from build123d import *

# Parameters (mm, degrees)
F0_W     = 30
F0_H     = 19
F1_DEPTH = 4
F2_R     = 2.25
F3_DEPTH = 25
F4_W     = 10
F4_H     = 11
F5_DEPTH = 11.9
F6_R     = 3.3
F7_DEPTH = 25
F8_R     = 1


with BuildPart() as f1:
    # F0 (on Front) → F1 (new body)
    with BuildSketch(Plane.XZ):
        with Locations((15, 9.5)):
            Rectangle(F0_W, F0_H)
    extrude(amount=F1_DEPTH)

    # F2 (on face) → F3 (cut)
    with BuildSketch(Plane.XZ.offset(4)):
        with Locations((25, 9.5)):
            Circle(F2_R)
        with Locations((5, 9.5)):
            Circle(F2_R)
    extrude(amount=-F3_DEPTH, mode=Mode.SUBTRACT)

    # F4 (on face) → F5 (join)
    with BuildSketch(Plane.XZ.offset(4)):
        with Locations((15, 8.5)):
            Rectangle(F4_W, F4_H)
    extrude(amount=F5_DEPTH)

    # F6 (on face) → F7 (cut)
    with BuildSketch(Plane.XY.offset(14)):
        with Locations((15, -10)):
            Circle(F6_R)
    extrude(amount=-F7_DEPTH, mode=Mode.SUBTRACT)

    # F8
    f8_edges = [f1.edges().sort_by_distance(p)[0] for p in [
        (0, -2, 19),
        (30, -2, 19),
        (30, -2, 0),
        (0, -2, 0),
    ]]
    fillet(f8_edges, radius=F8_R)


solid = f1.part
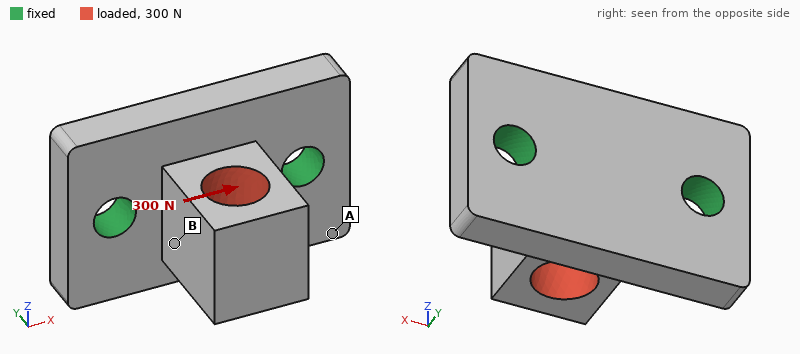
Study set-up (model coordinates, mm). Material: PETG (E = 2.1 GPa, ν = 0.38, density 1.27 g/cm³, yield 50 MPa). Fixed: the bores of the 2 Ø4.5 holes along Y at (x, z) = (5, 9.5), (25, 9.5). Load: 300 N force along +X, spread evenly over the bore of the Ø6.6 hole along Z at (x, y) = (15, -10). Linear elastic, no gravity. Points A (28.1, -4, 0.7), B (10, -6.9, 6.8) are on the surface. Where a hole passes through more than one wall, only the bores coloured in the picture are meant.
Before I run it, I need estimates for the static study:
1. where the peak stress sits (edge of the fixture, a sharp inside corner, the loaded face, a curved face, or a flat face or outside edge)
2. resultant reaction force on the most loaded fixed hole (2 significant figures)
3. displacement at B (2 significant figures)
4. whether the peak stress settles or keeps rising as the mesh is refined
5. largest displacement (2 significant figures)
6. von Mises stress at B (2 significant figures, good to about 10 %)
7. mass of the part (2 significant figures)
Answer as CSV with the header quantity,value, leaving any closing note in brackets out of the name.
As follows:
quantity,value
where the peak stress sits,edge of the fixture
resultant reaction force on the most loaded fixed hole,220 N
displacement at B,0.077 mm
whether the peak stress settles or keeps rising as the mesh is refined,keeps rising
largest displacement,0.26 mm
von Mises stress at B,15 MPa
mass of the part,3.9 g
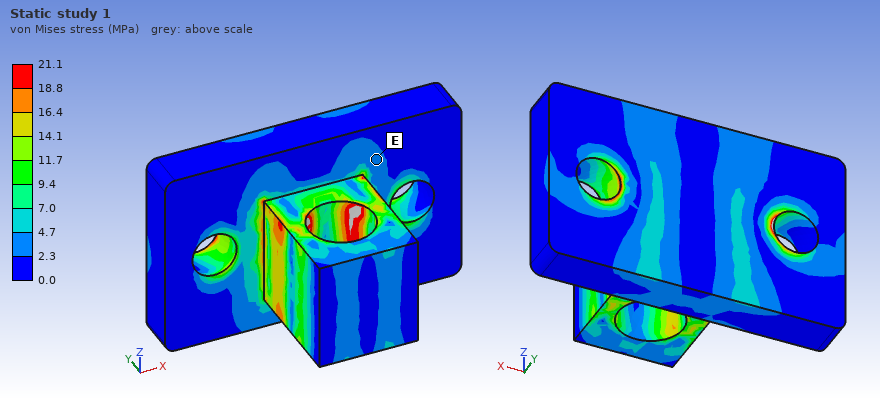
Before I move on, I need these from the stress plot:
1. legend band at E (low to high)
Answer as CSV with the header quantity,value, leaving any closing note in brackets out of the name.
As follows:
quantity,value
legend band at E,2.3 to 4.7 MPa
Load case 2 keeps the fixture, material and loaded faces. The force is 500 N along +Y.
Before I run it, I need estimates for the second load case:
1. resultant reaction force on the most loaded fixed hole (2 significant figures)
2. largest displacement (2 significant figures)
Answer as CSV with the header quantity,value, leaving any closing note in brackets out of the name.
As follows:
quantity,value
resultant reaction force on the most loaded fixed hole,260 N
largest displacement,0.14 mm
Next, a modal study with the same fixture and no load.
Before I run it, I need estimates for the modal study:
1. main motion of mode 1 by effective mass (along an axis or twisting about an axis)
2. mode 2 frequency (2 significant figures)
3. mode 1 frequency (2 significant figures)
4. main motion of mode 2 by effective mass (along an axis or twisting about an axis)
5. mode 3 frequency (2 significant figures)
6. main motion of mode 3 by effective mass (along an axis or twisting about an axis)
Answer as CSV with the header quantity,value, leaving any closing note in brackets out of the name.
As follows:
quantity,value
main motion of mode 1 by effective mass,along Z
mode 2 frequency,5500 Hz
mode 1 frequency,4100 Hz
main motion of mode 2 by effective mass,along X
mode 3 frequency,8300 Hz
main motion of mode 3 by effective mass,along Y
